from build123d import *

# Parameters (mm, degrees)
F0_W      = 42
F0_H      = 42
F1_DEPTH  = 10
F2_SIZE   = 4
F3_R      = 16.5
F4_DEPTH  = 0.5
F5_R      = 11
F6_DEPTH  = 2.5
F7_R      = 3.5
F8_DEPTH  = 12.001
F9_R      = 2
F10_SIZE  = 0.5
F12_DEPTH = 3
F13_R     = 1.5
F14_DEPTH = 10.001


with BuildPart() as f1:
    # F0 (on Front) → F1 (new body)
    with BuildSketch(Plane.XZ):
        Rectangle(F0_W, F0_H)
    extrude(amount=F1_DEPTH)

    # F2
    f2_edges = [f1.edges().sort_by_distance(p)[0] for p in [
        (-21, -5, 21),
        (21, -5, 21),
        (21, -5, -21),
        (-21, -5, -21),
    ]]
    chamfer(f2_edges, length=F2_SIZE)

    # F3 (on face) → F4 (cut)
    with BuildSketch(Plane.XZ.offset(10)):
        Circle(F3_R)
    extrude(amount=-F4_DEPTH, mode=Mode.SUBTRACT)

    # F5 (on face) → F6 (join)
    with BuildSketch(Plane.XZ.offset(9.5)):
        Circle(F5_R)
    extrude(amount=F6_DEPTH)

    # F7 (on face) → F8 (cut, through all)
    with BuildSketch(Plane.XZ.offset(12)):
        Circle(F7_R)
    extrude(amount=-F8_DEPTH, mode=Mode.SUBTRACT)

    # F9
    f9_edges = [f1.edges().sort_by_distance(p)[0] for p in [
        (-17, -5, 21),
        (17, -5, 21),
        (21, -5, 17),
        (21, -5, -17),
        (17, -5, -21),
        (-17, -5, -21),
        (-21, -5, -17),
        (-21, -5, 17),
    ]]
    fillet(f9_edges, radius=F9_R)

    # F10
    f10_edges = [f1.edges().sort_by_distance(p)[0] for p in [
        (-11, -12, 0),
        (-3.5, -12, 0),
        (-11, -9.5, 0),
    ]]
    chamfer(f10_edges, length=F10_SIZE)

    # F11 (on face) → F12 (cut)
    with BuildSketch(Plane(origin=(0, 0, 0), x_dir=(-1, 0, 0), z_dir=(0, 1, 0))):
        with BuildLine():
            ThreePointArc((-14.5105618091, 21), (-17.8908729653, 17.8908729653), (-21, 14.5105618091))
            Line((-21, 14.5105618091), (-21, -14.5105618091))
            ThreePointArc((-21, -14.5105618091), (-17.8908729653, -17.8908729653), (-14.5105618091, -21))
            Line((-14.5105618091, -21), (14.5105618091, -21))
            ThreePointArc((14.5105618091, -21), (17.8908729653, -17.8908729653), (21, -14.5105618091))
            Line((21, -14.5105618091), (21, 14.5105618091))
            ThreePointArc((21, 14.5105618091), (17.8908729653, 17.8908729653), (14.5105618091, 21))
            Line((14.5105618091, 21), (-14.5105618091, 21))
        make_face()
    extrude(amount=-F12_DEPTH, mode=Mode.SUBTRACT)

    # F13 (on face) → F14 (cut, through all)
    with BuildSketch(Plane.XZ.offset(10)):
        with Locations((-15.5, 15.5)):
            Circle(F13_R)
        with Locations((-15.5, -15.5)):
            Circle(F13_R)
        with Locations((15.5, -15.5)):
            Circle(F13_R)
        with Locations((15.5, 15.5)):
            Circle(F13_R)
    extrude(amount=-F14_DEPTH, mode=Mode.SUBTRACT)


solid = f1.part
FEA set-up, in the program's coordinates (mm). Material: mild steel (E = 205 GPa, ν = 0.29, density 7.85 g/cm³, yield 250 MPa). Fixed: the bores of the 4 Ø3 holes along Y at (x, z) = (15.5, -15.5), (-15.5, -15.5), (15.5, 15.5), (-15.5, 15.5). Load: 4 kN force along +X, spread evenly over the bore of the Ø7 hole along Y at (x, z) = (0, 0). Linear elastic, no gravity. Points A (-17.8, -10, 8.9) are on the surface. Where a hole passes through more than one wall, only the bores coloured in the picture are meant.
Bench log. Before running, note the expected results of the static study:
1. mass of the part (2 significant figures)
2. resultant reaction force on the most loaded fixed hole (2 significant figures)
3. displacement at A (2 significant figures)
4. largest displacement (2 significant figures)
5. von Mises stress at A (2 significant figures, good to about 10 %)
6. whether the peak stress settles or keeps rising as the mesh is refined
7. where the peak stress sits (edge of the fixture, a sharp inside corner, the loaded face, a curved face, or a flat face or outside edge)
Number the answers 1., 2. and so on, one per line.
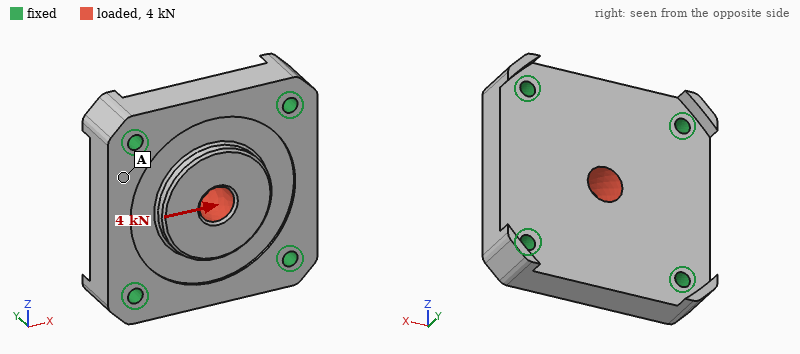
1. 96 g
2. 1.1 kN
3. 0.78 µm
4. 2.0 µm
5. 7.6 MPa
6. keeps rising
7. edge of the fixture
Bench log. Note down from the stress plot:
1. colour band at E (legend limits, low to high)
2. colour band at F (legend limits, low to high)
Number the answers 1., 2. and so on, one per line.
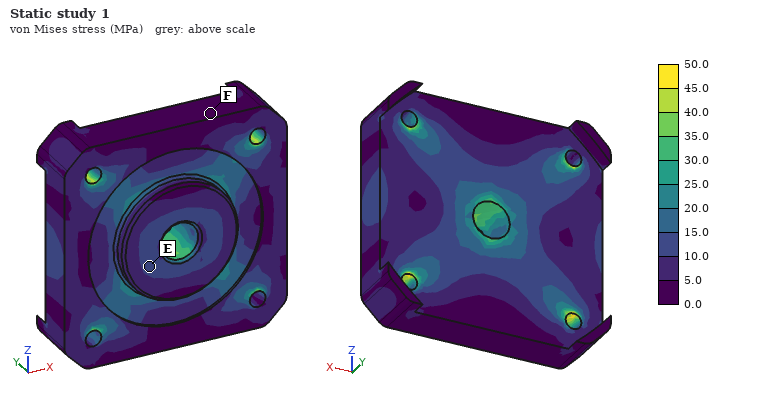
1. 10.0 to 15.0 MPa
2. 0.0 to 5.0 MPa
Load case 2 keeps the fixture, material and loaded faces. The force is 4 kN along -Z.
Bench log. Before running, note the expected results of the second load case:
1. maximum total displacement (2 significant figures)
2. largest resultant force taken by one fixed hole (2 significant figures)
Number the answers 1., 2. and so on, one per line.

1. 2.0 µm
2. 1.1 kN
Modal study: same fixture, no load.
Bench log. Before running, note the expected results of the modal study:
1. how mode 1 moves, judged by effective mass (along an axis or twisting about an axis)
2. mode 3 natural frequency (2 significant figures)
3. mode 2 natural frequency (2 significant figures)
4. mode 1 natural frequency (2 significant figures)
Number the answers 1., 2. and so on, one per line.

1. along Y
2. 30 kHz
3. 30 kHz
4. 21 kHz
